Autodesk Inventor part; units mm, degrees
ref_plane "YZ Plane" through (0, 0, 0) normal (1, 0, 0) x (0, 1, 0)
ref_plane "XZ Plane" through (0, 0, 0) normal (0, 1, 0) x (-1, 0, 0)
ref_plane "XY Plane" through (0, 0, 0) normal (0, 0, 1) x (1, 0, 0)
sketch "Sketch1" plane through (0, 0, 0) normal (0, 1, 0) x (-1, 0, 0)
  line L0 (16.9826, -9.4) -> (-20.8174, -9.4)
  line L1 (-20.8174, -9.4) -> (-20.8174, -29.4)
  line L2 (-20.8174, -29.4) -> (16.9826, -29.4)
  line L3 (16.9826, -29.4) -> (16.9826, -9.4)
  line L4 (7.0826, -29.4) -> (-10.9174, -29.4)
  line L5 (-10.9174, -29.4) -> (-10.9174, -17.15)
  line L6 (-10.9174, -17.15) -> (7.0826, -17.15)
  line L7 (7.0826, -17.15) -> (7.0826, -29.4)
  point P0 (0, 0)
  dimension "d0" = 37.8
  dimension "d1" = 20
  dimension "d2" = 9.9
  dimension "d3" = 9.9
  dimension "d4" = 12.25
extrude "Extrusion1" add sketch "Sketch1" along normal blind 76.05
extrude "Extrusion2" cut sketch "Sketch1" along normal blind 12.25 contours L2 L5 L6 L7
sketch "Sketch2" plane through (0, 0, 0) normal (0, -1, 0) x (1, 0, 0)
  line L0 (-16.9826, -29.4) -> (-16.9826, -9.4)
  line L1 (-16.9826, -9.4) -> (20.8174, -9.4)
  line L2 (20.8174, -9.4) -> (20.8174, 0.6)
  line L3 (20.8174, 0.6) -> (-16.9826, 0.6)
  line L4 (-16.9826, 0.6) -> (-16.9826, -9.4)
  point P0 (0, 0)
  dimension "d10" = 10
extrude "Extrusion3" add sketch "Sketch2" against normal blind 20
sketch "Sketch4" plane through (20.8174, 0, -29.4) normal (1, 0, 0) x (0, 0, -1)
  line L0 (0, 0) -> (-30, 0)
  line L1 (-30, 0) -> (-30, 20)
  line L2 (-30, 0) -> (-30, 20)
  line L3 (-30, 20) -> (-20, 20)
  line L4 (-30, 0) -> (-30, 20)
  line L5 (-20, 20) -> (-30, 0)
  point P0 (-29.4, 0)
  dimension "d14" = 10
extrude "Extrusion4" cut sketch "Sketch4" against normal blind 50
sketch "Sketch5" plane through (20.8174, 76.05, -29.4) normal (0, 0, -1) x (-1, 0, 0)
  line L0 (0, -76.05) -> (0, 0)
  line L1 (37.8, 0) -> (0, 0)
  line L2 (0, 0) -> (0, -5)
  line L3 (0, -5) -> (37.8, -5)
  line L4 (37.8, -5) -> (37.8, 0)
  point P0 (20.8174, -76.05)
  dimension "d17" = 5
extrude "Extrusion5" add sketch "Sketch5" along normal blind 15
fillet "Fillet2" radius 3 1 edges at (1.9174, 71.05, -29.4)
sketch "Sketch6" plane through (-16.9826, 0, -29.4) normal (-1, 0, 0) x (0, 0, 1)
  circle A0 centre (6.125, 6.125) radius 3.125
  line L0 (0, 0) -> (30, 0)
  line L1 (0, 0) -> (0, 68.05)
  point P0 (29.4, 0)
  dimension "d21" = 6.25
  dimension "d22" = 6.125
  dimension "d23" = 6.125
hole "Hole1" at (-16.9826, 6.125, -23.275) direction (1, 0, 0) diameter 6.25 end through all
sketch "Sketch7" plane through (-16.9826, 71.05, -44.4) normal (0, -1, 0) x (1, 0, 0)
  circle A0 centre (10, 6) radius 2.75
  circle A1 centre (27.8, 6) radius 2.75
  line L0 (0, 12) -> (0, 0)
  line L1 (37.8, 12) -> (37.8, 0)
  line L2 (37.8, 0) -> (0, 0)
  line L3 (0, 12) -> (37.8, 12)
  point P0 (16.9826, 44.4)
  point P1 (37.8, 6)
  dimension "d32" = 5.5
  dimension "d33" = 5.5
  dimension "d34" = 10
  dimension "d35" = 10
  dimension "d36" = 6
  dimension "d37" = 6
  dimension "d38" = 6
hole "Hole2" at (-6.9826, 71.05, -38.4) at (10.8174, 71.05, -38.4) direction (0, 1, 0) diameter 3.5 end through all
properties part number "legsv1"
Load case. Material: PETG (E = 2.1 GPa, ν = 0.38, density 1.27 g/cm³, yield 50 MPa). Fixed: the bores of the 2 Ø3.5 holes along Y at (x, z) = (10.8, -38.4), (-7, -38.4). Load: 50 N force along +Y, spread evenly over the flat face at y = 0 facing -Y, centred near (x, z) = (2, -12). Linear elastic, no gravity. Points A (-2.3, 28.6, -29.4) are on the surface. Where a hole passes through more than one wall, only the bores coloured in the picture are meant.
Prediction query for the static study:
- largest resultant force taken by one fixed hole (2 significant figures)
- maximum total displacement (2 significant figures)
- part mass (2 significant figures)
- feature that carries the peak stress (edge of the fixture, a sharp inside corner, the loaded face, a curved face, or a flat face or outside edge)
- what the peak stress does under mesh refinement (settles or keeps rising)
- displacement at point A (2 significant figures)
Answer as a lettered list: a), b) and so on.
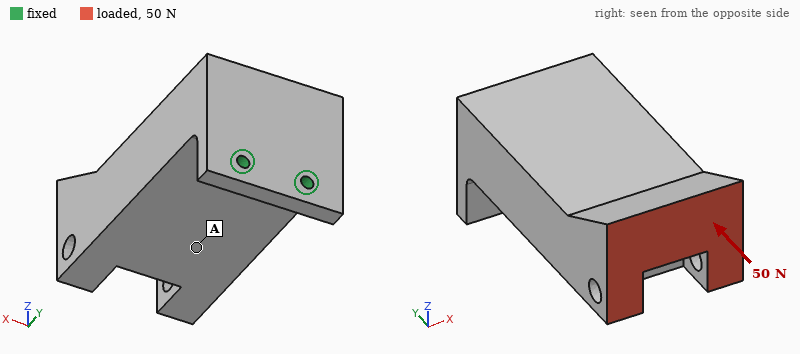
a) 25 N
b) 1.1 mm
c) 77 g
d) edge of the fixture
e) keeps rising
f) 0.61 mm
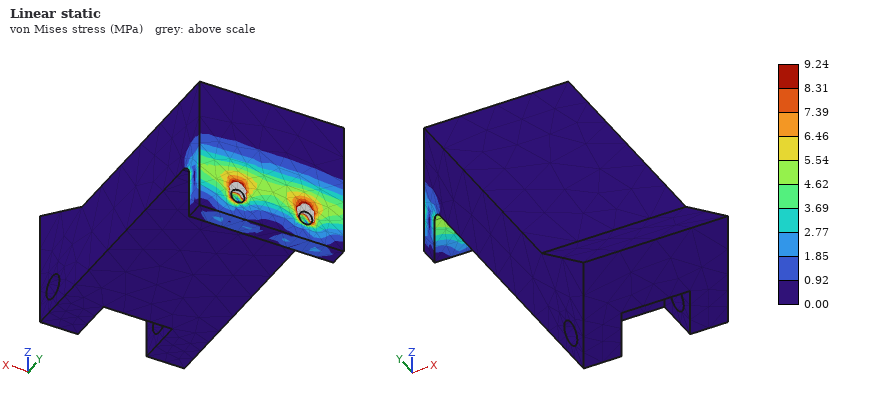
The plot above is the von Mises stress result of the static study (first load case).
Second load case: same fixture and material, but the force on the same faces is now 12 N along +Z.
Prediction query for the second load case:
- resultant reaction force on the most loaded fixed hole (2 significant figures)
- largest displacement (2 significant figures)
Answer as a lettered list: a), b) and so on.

a) 6.4 N
b) 0.93 mm
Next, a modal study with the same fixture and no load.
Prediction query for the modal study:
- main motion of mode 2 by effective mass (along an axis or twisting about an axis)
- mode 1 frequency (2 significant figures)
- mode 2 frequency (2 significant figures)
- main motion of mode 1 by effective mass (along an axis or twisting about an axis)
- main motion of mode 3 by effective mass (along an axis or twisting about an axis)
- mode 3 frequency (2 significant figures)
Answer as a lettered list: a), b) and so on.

a) along X
b) 120 Hz
c) 280 Hz
d) along Z
e) along Y
f) 1100 Hz
